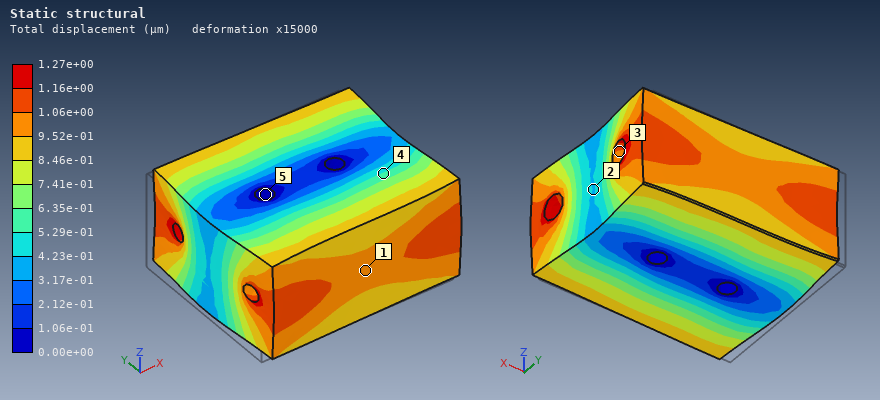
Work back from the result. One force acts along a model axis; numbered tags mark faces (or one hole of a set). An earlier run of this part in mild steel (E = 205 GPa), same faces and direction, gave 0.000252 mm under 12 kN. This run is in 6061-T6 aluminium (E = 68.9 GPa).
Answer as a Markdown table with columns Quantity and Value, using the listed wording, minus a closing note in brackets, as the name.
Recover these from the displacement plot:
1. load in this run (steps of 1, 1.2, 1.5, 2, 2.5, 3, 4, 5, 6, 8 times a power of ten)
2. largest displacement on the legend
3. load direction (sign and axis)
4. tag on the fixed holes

| Quantity | Value |
|---|---|
| load in this run | 20 kN |
| largest displacement on the legend | 1.27e+00 µm |
| load direction | +X |
| tag on the fixed holes | 5 |
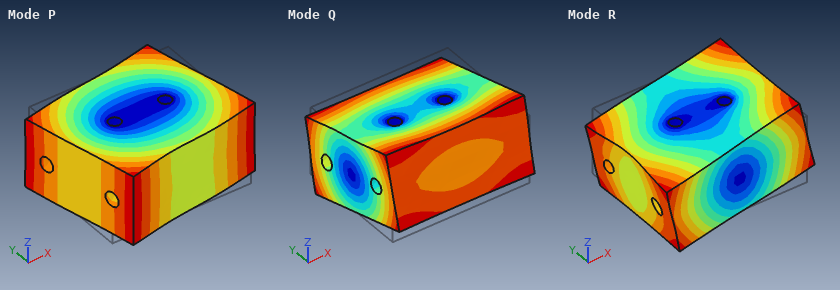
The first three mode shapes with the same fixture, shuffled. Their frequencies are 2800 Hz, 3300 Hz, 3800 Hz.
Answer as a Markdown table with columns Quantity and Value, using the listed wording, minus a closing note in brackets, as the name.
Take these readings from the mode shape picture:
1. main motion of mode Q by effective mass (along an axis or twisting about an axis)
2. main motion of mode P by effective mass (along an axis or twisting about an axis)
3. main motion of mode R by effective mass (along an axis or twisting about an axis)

| Quantity | Value |
|---|---|
| main motion of mode Q by effective mass | twisting about X |
| main motion of mode P by effective mass | twisting about Z |
| main motion of mode R by effective mass | twisting about Y |
